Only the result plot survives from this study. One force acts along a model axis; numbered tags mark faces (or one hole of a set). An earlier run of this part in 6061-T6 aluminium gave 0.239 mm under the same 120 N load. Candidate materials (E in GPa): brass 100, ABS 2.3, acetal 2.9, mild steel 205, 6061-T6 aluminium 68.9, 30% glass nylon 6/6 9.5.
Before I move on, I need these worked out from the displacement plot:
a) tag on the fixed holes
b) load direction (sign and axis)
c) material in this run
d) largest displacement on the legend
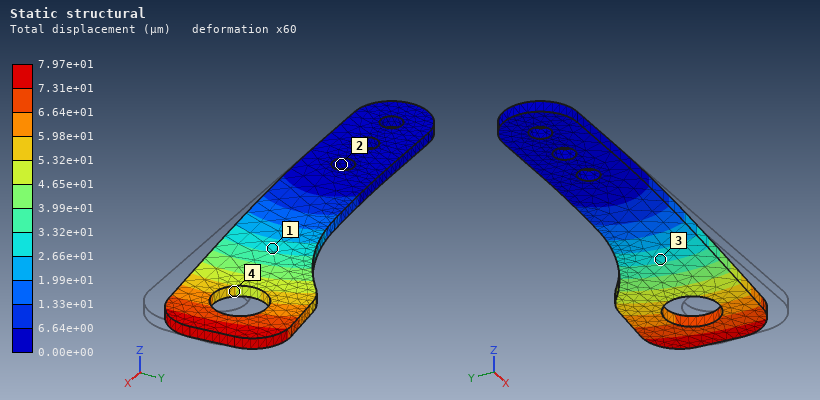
2
+Y
mild steel
7.97e+01 µm
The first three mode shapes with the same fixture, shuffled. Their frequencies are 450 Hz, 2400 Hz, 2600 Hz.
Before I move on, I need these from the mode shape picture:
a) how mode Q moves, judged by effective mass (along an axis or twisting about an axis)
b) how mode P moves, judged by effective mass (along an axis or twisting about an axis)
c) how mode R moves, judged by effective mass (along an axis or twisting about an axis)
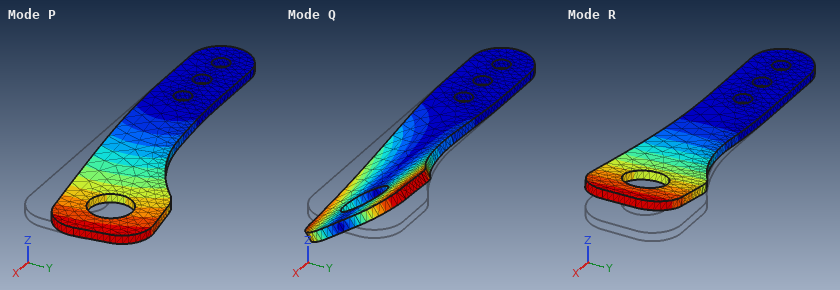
twisting about X
along Y
along Z
